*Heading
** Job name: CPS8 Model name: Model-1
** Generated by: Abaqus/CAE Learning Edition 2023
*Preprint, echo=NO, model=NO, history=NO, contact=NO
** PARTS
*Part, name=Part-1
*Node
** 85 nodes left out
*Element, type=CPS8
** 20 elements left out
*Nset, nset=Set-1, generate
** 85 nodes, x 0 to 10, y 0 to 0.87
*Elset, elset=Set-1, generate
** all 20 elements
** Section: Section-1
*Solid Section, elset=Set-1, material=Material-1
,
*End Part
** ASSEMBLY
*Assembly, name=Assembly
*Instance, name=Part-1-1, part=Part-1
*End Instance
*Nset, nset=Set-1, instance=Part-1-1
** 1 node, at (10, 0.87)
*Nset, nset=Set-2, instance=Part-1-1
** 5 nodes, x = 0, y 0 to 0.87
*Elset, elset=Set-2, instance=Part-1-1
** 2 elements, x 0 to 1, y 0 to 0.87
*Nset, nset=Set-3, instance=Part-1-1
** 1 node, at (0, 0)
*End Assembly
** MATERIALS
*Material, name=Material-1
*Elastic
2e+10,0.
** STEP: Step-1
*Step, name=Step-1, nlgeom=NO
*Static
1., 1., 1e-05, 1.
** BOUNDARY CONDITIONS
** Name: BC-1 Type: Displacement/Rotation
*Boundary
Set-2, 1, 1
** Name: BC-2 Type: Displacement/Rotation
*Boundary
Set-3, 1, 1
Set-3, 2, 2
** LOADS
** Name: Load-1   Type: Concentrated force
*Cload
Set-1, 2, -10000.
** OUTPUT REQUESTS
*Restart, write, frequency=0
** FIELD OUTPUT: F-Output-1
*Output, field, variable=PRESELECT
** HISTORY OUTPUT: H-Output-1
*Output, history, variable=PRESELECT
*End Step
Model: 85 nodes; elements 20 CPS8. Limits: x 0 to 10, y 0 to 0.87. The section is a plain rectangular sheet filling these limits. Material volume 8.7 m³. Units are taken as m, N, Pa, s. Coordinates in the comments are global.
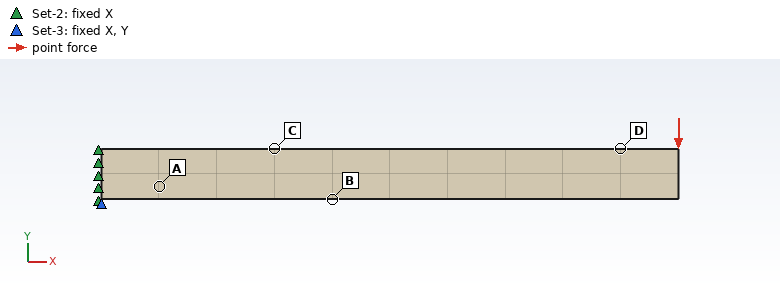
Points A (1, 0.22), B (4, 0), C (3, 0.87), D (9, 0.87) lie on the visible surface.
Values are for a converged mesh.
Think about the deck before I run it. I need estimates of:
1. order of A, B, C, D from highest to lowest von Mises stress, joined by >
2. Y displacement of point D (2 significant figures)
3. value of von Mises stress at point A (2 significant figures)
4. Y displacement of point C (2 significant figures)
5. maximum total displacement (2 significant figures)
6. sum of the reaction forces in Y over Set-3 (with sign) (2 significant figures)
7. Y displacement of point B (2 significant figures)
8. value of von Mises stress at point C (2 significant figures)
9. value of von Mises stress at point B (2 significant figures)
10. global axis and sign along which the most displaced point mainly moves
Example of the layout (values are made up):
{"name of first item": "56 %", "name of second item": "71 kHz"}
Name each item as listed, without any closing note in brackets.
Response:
{"order of A, B, C, D from highest to lowest von Mises stress, joined by >": "C > B > A > D", "Y displacement of point D": "-0.0026 m", "value of von Mises stress at point A": "3.6e+05 Pa", "Y displacement of point C": "-3.7e-04 m", "maximum total displacement": "0.0031 m", "sum of the reaction forces in Y over Set-3 (with sign)": "10000 N", "Y displacement of point B": "-6.4e-04 m", "value of von Mises stress at point C": "5.5e+05 Pa", "value of von Mises stress at point B": "4.8e+05 Pa", "global axis and sign along which the most displaced point mainly moves": "-Y"}
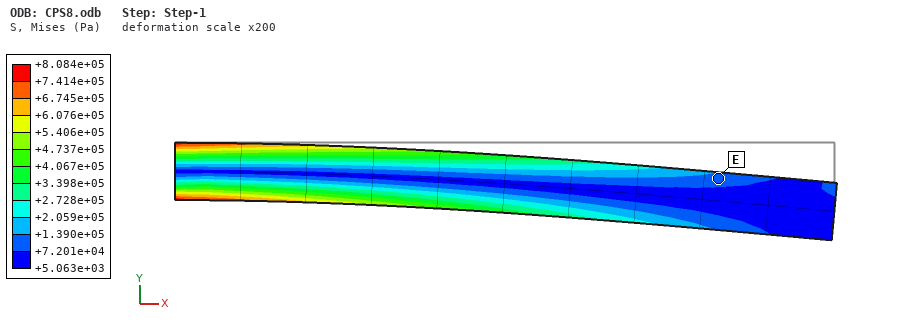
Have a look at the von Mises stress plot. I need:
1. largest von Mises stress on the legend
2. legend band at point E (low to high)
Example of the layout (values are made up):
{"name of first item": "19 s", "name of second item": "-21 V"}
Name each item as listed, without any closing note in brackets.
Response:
{"largest von Mises stress on the legend": "+8.084e+05 Pa", "legend band at point E": "+7.201e+04 to +1.390e+05 Pa"}
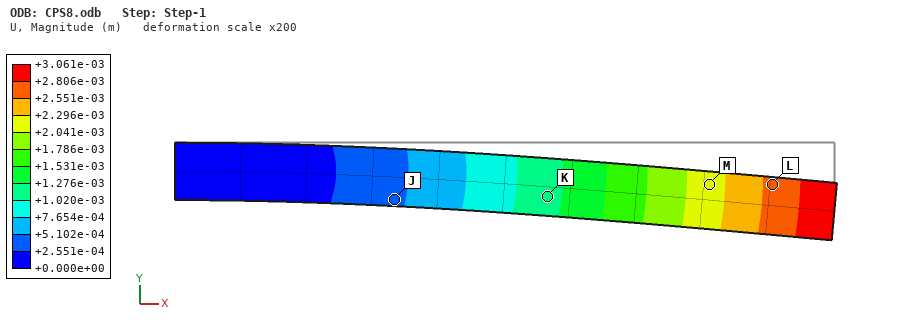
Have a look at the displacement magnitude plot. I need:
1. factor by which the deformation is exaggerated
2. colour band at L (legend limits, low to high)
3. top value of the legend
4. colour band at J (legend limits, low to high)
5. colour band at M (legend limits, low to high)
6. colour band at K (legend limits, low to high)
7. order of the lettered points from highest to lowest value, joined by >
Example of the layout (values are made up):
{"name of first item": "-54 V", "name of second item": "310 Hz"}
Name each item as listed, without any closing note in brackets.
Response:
{"factor by which the deformation is exaggerated": "200", "colour band at L": "+2.551e-03 to +2.806e-03 m", "top value of the legend": "+3.061e-03 m", "colour band at J": "+2.551e-04 to +5.102e-04 m", "colour band at M": "+2.041e-03 to +2.296e-03 m", "colour band at K": "+1.020e-03 to +1.276e-03 m", "order of the lettered points from highest to lowest value, joined by >": "L > M > K > J"}
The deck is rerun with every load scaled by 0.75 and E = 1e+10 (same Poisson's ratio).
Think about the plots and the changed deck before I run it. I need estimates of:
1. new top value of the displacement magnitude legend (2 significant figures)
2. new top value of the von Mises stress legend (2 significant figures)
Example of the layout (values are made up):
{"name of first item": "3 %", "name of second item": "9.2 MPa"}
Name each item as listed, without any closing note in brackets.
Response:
{"new top value of the displacement magnitude legend": "0.0046 m", "new top value of the von Mises stress legend": "6.1e+05 Pa"}
